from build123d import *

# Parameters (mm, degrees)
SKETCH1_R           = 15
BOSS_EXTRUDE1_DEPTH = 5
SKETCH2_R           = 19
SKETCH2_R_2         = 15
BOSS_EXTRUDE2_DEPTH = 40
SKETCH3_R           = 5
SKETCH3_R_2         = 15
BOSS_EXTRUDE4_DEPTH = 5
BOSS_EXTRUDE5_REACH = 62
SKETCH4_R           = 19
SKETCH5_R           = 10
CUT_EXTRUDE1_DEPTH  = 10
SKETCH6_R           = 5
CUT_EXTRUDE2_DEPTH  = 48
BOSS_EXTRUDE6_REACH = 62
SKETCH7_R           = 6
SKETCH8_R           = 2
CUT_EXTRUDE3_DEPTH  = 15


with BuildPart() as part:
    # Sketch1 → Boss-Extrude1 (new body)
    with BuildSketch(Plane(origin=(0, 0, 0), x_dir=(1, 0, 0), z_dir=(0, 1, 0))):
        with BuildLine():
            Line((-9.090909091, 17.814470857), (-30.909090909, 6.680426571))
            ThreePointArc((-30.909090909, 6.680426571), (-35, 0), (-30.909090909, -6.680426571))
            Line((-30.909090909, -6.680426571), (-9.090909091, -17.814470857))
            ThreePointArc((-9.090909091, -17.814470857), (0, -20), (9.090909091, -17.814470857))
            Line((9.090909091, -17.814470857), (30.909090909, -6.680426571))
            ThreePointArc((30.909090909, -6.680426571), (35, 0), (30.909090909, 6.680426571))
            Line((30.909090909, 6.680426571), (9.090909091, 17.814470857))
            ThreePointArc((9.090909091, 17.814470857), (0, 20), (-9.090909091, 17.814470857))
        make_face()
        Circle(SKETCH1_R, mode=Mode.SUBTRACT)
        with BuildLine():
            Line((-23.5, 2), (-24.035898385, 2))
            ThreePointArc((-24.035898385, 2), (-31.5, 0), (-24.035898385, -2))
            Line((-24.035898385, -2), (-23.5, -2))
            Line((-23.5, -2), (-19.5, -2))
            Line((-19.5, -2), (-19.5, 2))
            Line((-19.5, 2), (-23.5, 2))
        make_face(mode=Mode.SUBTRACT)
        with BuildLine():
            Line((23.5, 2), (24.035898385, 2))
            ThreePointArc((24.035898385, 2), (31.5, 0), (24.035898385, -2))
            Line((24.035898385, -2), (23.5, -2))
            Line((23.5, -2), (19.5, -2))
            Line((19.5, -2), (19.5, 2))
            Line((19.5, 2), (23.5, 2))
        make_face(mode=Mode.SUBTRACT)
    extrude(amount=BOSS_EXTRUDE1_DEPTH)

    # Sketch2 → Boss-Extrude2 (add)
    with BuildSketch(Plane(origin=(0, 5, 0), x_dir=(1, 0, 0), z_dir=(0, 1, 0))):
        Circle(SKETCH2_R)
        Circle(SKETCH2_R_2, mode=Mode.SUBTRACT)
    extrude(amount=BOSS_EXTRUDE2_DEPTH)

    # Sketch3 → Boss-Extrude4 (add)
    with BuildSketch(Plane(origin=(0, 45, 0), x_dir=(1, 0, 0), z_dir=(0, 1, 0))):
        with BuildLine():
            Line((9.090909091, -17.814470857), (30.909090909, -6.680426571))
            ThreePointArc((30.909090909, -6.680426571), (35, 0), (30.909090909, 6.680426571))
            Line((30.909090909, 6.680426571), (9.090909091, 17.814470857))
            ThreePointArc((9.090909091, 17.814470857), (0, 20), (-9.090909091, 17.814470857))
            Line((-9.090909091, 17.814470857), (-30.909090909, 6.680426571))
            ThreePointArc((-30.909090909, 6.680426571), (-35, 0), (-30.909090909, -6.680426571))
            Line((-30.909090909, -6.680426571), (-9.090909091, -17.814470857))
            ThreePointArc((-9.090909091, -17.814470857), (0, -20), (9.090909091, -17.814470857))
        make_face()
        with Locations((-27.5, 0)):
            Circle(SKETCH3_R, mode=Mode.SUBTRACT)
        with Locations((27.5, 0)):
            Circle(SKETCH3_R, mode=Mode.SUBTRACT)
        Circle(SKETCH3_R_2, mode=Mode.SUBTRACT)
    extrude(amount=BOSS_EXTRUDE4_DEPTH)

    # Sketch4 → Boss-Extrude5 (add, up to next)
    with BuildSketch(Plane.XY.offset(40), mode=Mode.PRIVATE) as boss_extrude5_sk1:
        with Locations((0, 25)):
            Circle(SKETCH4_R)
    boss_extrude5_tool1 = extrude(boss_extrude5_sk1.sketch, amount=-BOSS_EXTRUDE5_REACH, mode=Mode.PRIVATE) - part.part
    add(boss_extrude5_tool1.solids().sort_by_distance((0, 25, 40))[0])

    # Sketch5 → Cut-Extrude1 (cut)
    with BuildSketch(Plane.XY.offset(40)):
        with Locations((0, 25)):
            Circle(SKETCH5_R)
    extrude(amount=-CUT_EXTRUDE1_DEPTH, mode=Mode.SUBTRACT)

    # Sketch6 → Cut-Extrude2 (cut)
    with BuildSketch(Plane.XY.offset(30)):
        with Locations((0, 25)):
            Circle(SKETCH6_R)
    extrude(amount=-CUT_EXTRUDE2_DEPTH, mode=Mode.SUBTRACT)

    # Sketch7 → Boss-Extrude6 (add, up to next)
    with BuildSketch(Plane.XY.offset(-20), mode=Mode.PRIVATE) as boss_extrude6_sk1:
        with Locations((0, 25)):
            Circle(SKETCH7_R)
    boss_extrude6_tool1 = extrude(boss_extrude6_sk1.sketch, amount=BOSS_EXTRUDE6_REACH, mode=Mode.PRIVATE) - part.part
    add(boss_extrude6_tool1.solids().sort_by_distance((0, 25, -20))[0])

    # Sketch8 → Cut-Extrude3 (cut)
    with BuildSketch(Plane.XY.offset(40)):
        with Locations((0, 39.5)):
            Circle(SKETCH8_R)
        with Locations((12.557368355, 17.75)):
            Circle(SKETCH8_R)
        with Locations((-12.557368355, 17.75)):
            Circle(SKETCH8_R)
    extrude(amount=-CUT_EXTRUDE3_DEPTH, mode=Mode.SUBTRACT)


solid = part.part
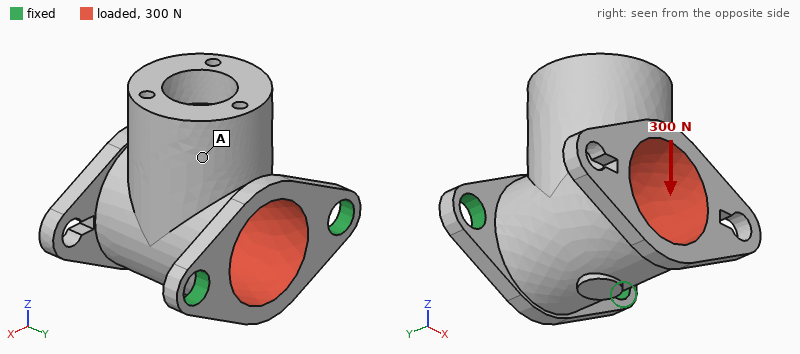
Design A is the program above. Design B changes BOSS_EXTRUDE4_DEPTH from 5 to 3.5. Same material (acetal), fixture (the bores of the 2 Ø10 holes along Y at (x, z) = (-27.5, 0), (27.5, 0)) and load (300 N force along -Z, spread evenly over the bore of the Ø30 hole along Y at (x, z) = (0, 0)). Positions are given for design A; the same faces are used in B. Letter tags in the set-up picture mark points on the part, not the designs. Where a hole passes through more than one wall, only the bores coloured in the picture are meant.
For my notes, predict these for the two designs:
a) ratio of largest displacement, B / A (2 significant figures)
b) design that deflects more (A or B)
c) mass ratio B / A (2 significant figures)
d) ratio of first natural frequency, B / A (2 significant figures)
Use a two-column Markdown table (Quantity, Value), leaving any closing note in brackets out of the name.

| Quantity | Value |
|---|---|
| ratio of largest displacement, B / A | 1.9 |
| design that deflects more | B |
| mass ratio B / A | 0.97 |
| ratio of first natural frequency, B / A | 0.73 |
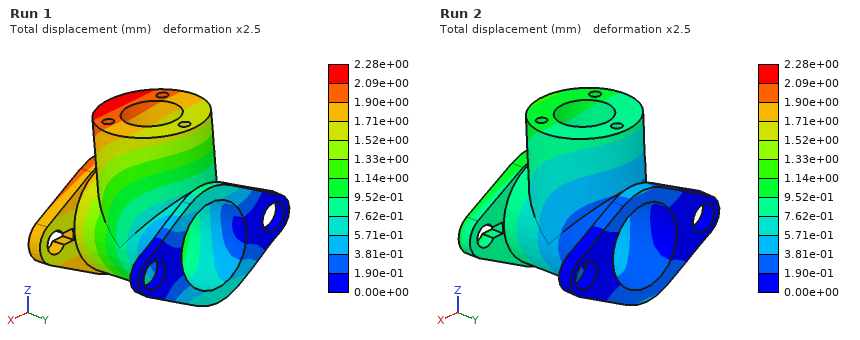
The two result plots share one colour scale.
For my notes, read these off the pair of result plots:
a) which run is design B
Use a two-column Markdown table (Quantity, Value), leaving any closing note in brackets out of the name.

| Quantity | Value |
|---|---|
| which run is design B | Run 1 |
